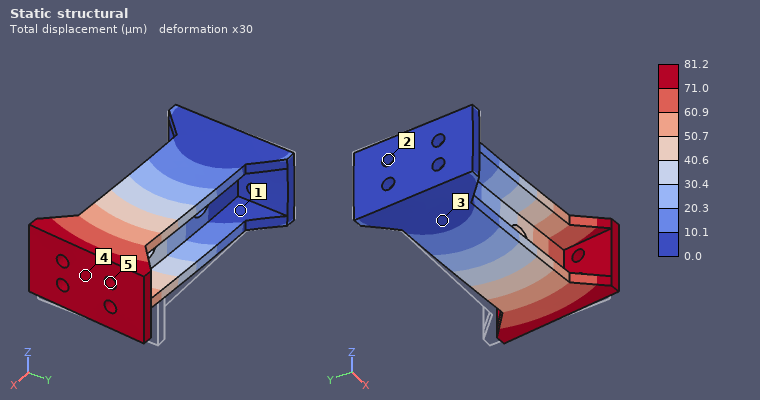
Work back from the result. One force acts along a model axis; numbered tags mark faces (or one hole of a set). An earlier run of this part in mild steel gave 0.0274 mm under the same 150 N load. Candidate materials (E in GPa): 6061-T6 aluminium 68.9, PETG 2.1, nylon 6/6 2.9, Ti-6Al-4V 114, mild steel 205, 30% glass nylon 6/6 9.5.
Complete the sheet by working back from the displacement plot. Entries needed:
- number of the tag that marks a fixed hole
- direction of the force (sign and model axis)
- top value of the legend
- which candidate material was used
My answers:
2
-Y
81.2 µm
6061-T6 aluminium
